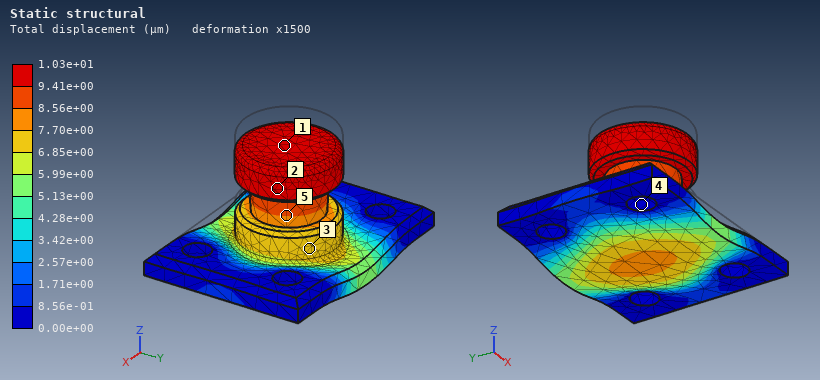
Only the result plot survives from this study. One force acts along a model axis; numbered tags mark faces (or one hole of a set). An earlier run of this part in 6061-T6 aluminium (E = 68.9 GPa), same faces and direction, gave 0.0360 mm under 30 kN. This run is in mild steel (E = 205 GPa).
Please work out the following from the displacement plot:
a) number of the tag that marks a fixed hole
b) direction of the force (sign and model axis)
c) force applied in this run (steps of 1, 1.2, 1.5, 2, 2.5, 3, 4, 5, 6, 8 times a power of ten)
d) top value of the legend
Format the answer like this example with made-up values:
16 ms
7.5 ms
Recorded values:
4
-Z
25 kN
1.03e+01 µm
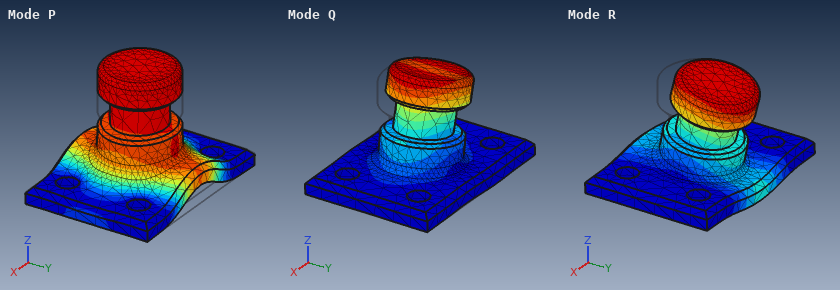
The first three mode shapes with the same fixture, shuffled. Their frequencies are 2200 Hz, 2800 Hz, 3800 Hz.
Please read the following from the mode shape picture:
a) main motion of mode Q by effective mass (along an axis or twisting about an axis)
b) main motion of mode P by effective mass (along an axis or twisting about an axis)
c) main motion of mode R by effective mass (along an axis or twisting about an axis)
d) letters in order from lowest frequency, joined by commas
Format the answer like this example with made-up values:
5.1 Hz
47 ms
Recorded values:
along X
along Z
along Y
R, Q, P
